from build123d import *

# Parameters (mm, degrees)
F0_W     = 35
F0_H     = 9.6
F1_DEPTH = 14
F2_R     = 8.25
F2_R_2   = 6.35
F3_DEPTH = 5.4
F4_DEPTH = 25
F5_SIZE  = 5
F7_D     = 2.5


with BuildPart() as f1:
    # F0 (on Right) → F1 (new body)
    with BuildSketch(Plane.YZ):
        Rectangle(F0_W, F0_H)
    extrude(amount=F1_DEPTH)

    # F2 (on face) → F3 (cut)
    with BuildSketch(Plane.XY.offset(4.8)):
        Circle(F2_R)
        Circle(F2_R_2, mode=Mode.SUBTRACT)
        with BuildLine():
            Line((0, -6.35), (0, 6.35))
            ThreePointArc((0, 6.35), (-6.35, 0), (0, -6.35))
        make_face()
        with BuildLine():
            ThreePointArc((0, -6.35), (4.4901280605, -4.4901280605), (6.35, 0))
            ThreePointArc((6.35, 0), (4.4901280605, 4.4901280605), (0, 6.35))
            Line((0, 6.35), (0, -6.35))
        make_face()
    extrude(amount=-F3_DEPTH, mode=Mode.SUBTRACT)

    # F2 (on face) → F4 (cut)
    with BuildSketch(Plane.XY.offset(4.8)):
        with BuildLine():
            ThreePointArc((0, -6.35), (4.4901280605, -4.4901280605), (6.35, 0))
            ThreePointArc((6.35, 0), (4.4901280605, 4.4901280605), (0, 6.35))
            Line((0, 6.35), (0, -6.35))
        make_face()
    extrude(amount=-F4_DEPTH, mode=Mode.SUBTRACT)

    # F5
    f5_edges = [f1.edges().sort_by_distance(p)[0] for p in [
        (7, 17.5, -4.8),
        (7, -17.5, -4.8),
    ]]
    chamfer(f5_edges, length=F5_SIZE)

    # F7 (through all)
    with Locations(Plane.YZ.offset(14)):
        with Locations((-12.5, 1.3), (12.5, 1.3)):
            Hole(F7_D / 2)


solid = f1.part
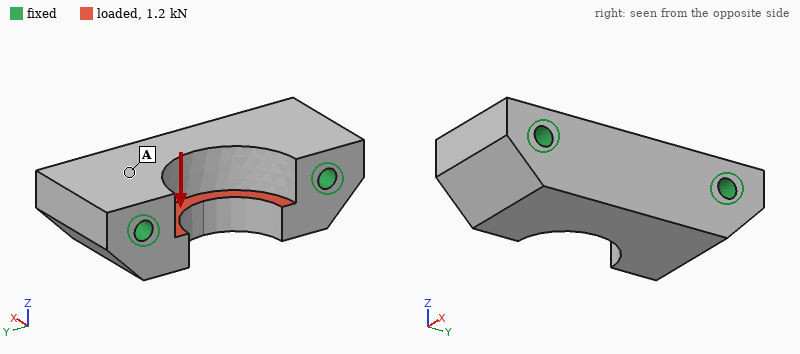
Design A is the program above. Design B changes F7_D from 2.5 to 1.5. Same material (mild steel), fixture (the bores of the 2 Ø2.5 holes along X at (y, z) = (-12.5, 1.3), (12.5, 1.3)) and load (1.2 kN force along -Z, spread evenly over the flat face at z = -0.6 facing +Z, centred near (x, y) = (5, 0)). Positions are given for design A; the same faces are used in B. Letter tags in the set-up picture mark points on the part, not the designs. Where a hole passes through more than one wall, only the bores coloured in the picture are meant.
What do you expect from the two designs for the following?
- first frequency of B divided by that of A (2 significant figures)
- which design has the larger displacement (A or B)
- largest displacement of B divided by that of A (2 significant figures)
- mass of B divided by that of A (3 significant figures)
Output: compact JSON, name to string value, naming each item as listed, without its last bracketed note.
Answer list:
{"first frequency of B divided by that of A": "0.83", "which design has the larger displacement": "B", "largest displacement of B divided by that of A": "1.2", "mass of B divided by that of A": "1.03"}
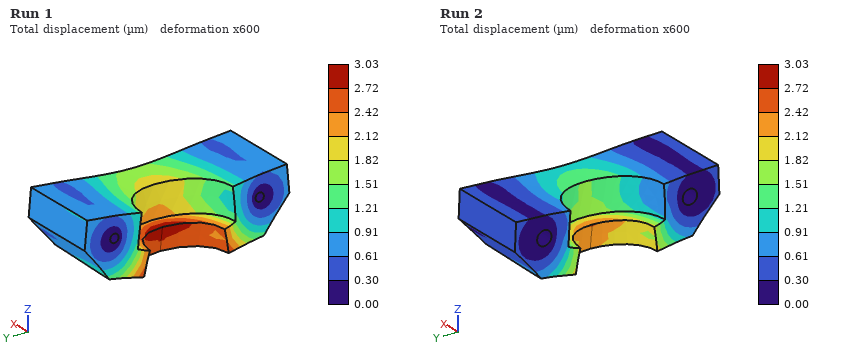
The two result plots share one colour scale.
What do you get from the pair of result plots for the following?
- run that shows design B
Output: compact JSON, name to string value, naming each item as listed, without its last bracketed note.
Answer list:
{"run that shows design B": "Run 1"}
